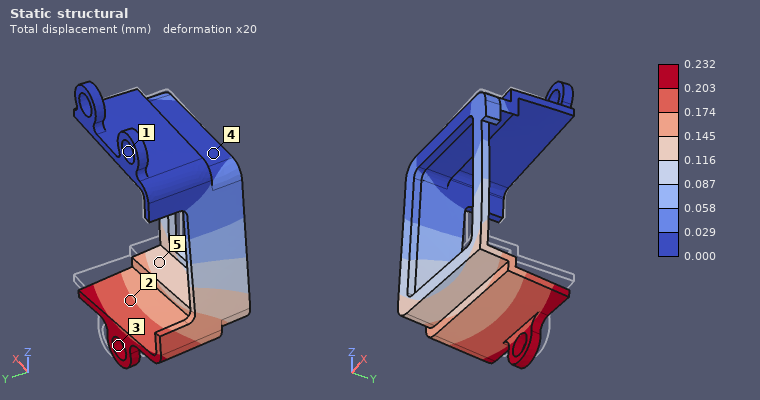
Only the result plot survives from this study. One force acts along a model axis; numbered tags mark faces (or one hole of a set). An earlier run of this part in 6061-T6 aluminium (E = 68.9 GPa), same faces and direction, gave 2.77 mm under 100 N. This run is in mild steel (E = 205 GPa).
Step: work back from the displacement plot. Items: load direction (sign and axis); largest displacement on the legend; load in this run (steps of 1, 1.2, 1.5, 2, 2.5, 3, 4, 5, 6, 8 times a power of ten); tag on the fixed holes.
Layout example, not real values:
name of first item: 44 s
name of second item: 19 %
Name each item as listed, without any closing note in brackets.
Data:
load direction: -X
largest displacement on the legend: 0.232 mm
load in this run: 25 N
tag on the fixed holes: 1
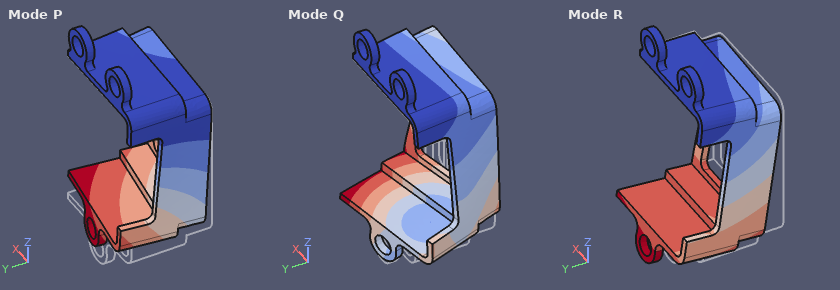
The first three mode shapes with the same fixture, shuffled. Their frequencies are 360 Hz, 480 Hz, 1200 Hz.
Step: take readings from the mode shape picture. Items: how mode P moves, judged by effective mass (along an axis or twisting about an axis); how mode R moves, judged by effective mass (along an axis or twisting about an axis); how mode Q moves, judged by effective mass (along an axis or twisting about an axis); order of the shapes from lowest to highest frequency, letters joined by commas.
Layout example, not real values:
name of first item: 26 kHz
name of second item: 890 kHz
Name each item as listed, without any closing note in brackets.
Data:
how mode P moves, judged by effective mass: along X
how mode R moves, judged by effective mass: along Y
how mode Q moves, judged by effective mass: along Z
order of the shapes from lowest to highest frequency, letters joined by commas: R, P, Q
